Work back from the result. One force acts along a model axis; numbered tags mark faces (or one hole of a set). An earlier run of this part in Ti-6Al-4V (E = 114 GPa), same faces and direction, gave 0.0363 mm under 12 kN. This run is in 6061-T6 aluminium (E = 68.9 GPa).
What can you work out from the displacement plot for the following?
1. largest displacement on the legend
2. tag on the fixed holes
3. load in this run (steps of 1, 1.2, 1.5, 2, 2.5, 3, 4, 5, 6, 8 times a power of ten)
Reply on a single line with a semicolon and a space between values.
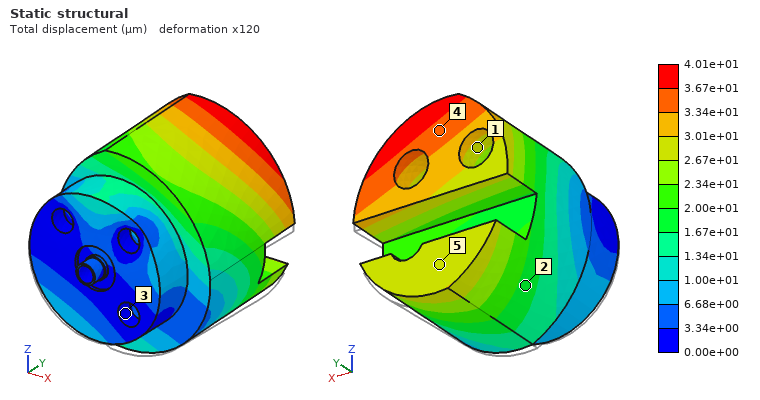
4.01e+01 µm; 3; 8 kN
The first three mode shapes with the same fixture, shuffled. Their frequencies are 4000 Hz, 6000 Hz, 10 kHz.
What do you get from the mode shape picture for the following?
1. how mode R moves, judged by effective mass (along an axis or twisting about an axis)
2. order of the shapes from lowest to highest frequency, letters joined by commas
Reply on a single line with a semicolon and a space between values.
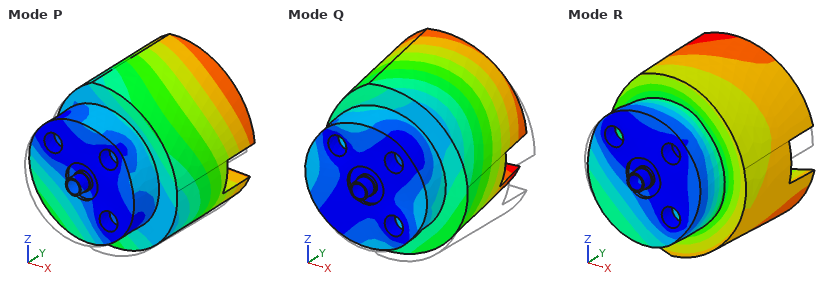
twisting about Y; P, Q, R
